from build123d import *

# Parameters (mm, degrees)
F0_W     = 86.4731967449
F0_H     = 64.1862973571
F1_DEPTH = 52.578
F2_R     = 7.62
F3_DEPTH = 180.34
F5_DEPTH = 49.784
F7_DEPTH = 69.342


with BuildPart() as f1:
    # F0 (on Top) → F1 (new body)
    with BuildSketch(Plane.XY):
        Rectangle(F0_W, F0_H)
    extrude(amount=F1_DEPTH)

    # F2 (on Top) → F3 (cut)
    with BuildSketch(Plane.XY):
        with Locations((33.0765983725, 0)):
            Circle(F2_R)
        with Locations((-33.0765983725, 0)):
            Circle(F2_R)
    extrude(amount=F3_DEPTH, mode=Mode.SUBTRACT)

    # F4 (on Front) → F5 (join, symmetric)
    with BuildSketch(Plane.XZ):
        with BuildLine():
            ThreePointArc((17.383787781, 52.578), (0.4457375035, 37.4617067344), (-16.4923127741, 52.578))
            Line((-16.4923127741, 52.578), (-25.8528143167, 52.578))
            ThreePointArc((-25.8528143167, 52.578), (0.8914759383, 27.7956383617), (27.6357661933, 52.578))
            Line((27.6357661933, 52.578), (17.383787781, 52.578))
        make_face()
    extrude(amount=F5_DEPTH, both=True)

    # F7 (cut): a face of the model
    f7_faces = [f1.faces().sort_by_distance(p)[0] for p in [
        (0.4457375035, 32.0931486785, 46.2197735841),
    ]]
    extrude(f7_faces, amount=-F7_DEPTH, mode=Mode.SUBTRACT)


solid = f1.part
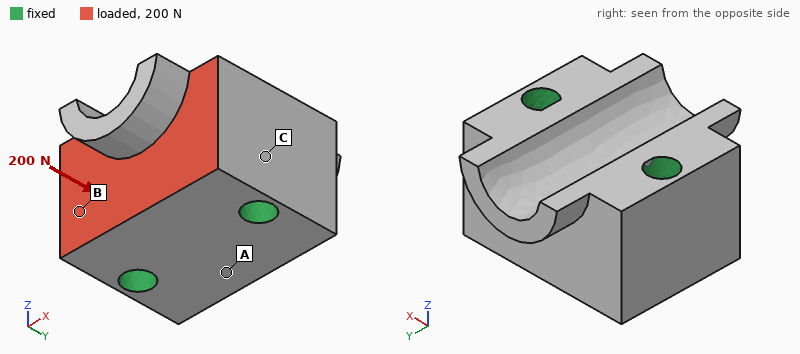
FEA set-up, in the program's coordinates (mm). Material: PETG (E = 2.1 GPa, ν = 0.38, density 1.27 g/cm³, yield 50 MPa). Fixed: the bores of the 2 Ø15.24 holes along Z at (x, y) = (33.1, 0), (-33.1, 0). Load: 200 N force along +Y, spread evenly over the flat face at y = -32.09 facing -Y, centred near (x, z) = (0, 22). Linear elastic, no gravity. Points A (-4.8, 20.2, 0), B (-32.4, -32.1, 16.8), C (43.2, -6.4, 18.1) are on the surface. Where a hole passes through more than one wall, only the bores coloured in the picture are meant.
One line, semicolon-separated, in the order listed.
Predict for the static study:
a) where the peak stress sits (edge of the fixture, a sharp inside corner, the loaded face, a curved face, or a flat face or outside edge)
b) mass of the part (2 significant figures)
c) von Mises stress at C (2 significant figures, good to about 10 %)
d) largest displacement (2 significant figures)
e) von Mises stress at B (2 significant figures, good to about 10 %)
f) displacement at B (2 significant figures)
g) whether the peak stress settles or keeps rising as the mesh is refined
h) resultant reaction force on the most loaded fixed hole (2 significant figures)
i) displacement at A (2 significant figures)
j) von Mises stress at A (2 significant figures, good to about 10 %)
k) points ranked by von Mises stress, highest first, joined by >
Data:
edge of the fixture; 340 g; 0.040 MPa; 1.5 µm; 0.061 MPa; 0.80 µm; keeps rising; 100 N; 0.57 µm; 0.015 MPa; B > C > A
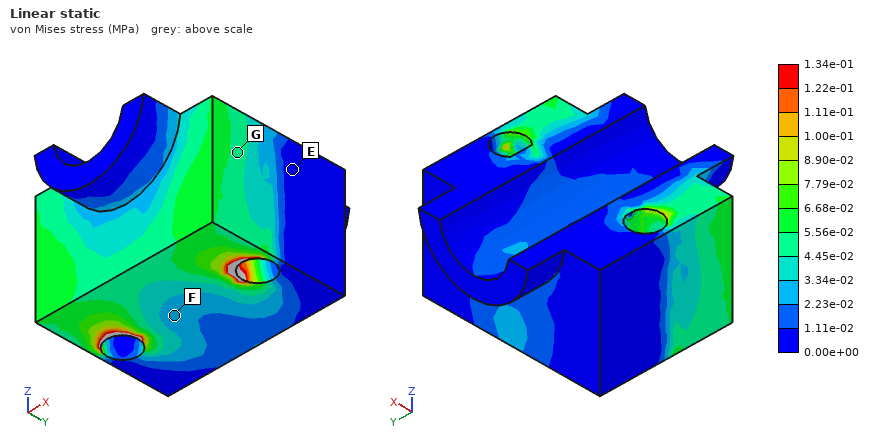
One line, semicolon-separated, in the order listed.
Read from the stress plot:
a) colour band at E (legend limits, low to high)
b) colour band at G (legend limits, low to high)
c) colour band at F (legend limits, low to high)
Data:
0.00e+00 to 1.11e-02 MPa; 4.45e-02 to 5.56e-02 MPa; 2.23e-02 to 3.34e-02 MPa
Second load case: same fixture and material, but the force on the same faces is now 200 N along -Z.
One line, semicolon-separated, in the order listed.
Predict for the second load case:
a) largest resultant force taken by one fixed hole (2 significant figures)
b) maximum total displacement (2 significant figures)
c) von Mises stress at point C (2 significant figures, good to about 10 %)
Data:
100 N; 4.8 µm; 0.052 MPa
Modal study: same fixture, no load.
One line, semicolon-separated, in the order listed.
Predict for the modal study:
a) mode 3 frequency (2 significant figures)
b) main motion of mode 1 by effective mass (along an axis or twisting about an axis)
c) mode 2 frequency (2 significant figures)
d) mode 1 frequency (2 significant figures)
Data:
3900 Hz; twisting about X; 3700 Hz; 3600 Hz
